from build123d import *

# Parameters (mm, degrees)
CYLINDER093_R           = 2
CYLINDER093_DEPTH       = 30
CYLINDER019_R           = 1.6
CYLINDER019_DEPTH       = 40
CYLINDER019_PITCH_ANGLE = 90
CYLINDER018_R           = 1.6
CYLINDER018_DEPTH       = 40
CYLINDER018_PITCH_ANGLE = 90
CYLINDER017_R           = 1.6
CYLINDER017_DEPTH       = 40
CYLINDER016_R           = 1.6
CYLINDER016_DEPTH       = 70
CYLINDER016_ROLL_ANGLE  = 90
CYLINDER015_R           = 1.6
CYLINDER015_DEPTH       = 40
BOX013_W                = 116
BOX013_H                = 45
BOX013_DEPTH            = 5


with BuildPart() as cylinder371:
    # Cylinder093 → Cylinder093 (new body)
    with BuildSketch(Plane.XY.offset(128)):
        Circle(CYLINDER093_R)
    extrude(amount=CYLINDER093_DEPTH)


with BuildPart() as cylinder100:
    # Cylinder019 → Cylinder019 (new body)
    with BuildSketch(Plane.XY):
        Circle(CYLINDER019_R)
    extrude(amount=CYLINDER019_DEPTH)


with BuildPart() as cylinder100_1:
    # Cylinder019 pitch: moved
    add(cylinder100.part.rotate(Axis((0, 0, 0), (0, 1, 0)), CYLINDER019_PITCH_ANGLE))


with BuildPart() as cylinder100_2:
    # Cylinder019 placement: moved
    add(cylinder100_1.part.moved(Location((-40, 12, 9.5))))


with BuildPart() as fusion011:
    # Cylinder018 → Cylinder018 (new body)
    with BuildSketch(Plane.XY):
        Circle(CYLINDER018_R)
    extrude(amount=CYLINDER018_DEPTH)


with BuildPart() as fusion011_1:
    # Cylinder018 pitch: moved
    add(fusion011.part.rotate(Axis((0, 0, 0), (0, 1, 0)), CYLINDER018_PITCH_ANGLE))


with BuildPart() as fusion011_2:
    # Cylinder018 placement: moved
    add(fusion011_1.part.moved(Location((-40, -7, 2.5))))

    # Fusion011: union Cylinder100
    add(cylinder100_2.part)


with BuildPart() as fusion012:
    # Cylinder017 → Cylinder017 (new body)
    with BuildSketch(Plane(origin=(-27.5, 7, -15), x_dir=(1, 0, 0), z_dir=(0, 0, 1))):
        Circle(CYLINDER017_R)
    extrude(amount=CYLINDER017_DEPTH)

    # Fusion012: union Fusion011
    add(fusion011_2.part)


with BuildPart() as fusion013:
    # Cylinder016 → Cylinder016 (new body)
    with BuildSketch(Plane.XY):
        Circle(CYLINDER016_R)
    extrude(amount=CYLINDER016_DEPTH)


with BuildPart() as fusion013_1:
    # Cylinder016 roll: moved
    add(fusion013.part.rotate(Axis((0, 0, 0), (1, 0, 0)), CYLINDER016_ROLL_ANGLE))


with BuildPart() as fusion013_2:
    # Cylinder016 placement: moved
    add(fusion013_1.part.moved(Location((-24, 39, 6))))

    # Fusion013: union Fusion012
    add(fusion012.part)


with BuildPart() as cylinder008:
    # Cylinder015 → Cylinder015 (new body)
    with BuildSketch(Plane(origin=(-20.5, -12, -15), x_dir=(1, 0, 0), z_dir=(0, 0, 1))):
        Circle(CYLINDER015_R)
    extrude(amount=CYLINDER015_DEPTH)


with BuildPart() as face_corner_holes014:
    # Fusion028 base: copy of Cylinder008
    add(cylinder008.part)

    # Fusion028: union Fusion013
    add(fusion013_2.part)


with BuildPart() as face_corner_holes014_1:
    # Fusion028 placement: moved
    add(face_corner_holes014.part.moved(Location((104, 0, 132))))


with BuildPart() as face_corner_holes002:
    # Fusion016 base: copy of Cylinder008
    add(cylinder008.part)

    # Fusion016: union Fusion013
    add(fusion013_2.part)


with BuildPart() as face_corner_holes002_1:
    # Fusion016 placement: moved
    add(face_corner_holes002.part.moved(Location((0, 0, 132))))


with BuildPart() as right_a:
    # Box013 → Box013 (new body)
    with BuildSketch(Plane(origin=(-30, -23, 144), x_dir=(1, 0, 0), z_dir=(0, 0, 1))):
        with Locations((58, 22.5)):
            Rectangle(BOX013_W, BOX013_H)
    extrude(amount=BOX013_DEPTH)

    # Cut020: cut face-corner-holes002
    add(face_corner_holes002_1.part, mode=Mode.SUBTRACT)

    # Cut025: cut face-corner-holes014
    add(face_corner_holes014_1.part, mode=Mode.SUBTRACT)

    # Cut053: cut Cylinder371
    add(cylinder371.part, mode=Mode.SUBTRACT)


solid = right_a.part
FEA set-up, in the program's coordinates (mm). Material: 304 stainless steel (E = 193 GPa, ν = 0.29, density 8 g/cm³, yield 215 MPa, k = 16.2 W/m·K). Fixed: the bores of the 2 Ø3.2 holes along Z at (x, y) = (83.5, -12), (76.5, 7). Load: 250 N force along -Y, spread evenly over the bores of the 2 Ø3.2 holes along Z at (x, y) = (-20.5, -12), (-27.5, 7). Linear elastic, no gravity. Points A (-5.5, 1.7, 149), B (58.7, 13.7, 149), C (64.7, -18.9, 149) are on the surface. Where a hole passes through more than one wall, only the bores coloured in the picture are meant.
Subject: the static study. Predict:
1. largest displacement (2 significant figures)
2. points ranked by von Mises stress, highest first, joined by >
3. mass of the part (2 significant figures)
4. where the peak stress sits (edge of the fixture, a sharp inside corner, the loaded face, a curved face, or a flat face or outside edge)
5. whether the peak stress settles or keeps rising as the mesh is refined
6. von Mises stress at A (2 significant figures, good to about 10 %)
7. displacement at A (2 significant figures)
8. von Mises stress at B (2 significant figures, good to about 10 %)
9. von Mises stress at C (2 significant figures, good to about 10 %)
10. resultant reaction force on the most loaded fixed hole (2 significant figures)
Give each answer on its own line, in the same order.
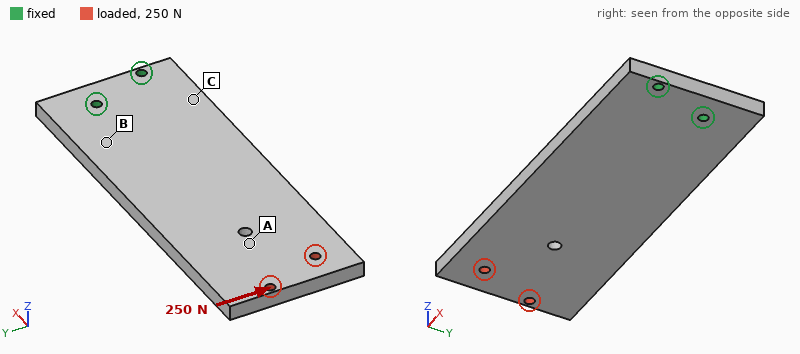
26 µm
C > B > A
210 g
edge of the fixture
keeps rising
3.2 MPa
18 µm
7.8 MPa
12 MPa
1.2 kN
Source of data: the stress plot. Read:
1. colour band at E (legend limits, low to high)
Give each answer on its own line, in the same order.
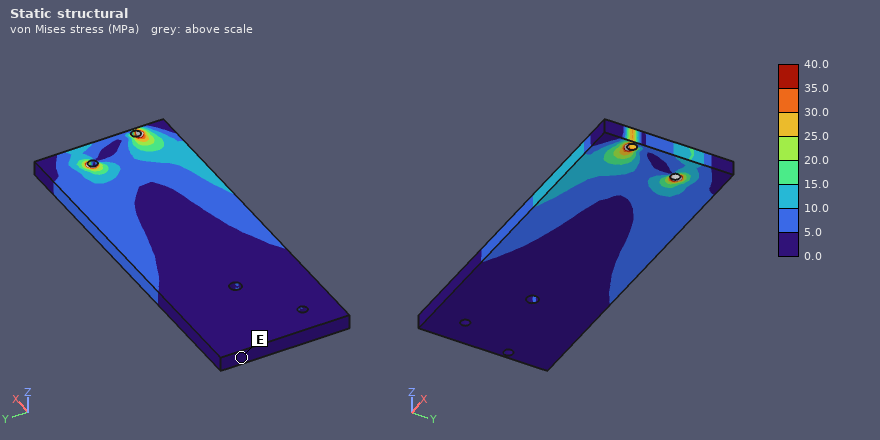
0.0 to 5.0 MPa
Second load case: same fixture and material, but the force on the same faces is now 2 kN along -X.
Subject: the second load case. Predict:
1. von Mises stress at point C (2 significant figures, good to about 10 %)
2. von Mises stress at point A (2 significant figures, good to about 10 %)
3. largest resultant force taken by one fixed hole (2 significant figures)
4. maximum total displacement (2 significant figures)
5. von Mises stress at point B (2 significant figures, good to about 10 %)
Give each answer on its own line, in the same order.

9.7 MPa
8.8 MPa
1.0 kN
8.1 µm
7.7 MPa
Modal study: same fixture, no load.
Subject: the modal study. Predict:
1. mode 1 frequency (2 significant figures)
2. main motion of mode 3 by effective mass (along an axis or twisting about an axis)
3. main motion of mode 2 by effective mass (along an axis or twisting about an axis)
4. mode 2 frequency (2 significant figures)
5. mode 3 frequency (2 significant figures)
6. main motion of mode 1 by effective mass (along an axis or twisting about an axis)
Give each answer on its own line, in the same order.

330 Hz
along Y
twisting about X
1600 Hz
2000 Hz
along Z
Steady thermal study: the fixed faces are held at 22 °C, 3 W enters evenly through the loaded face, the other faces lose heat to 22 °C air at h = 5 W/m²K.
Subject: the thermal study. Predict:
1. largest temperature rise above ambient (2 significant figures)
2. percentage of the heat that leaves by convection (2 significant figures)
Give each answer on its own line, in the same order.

63 K
51 %
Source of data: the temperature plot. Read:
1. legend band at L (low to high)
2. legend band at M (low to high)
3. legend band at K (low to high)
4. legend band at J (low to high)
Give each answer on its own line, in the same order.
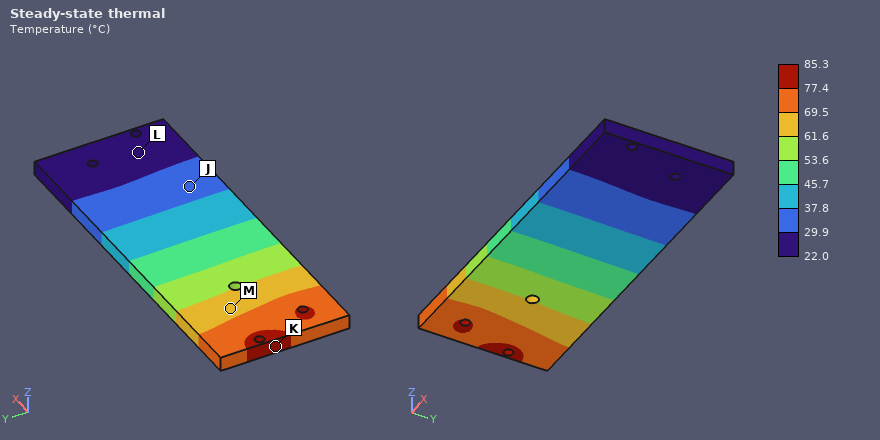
22.0 to 29.9 °C
61.6 to 69.5 °C
77.4 to 85.3 °C
29.9 to 37.8 °C
